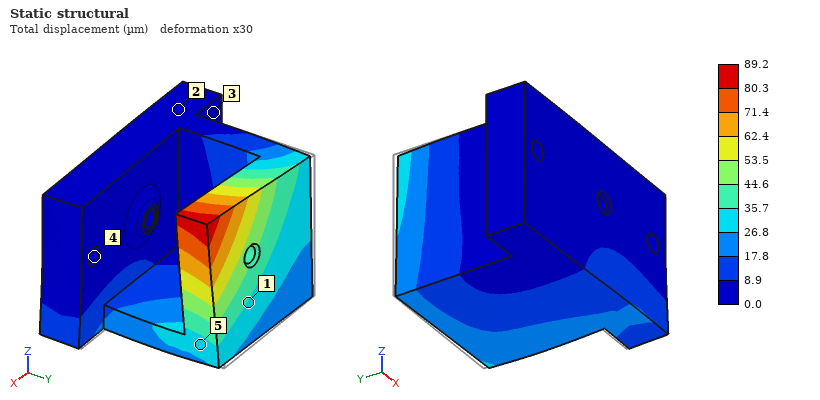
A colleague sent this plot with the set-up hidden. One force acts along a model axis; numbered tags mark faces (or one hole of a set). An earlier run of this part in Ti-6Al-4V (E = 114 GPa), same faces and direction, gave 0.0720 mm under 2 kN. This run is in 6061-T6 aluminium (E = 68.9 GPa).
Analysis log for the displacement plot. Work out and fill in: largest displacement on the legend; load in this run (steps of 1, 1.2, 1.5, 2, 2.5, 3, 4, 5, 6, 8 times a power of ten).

89.2 µm
1.5 kN
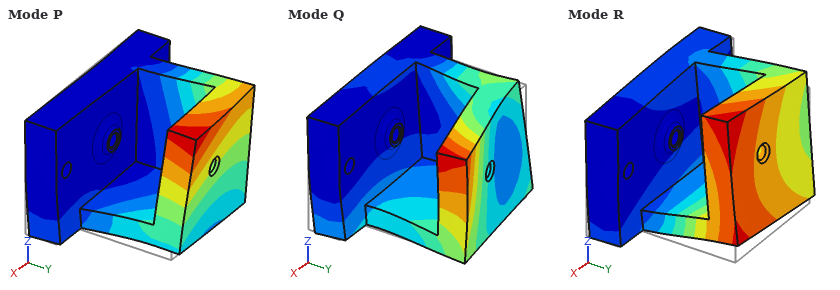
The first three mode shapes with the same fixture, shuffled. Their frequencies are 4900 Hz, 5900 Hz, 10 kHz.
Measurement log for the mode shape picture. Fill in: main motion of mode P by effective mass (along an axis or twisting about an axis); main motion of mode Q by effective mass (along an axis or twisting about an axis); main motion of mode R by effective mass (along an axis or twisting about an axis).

along X
along Y
along Z
